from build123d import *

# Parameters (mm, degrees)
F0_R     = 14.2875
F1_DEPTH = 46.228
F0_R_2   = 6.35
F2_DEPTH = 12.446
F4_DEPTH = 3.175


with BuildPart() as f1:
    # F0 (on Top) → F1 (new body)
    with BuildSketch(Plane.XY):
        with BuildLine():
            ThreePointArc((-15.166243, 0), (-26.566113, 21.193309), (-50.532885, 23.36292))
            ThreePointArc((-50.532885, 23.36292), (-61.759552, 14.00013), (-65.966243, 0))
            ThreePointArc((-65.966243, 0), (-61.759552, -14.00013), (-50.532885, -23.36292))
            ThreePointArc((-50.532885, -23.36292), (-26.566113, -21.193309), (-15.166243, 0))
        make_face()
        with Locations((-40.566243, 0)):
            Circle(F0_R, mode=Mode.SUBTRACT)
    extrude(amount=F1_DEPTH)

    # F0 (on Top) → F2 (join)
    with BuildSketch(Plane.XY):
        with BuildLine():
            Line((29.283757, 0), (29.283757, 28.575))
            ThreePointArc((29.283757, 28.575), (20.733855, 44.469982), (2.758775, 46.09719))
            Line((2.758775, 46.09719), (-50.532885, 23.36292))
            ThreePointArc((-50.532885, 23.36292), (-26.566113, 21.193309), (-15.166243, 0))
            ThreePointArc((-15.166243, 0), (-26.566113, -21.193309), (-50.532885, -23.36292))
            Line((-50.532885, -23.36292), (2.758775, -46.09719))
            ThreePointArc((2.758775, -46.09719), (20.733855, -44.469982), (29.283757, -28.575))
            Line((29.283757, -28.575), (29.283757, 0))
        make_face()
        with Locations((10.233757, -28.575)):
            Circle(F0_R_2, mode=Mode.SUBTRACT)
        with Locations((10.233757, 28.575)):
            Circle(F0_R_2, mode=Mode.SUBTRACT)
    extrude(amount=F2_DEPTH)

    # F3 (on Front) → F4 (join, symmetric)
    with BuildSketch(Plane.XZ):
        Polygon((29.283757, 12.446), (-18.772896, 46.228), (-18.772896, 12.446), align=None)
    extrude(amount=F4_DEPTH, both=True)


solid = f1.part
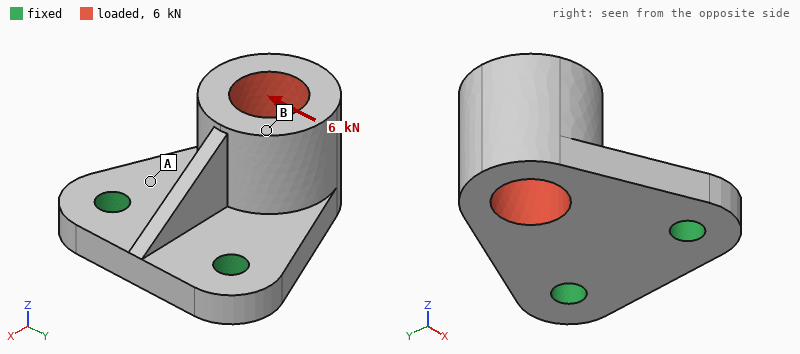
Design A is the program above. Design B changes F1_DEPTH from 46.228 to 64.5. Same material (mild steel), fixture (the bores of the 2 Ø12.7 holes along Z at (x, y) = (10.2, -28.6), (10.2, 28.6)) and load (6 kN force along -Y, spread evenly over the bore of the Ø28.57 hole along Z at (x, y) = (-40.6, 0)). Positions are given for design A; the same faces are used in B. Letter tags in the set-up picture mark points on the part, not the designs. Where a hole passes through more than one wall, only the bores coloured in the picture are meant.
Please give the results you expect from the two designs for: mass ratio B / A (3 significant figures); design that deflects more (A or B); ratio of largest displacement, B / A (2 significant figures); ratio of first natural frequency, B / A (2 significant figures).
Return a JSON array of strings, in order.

["1.21", "B", "1.9", "0.78"]
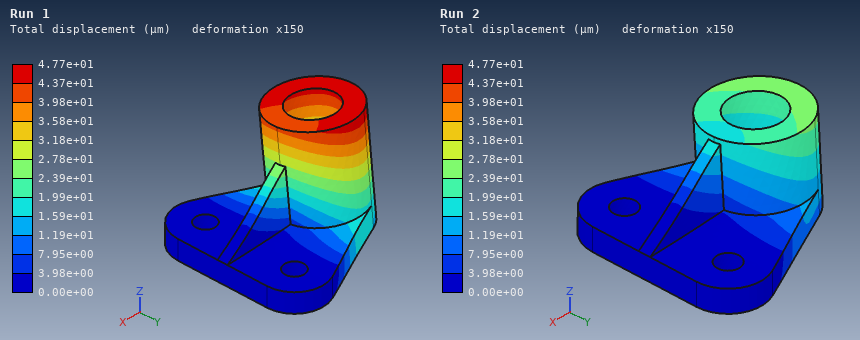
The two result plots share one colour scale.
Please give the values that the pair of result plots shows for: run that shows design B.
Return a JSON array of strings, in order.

["Run 1"]
